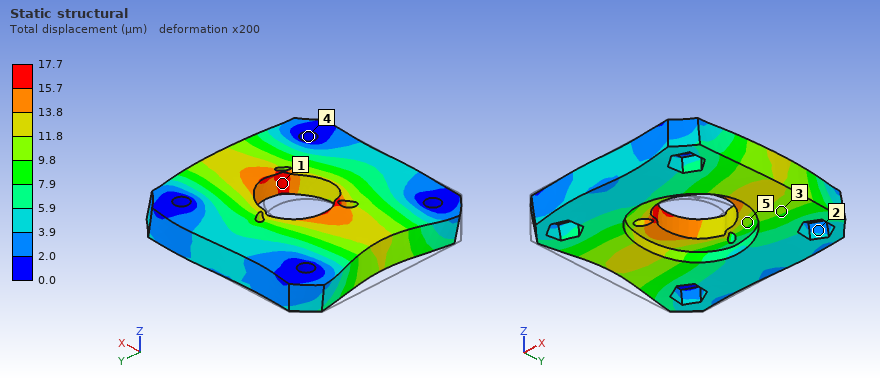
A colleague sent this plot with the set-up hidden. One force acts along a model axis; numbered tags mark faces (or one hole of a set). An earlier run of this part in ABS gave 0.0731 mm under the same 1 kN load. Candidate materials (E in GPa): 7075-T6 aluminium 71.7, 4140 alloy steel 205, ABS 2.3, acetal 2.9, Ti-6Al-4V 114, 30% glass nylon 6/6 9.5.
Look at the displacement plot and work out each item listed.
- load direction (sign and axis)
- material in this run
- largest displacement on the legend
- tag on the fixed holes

+X
30% glass nylon 6/6
17.7 µm
4
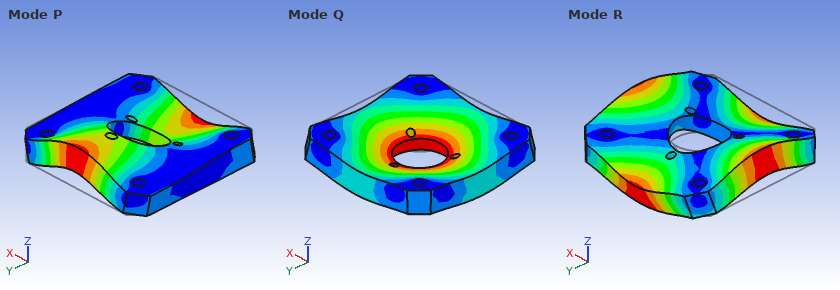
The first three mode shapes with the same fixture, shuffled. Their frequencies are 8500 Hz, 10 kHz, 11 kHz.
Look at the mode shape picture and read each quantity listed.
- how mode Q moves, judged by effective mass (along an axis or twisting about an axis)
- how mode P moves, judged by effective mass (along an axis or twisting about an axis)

along Z
twisting about X
